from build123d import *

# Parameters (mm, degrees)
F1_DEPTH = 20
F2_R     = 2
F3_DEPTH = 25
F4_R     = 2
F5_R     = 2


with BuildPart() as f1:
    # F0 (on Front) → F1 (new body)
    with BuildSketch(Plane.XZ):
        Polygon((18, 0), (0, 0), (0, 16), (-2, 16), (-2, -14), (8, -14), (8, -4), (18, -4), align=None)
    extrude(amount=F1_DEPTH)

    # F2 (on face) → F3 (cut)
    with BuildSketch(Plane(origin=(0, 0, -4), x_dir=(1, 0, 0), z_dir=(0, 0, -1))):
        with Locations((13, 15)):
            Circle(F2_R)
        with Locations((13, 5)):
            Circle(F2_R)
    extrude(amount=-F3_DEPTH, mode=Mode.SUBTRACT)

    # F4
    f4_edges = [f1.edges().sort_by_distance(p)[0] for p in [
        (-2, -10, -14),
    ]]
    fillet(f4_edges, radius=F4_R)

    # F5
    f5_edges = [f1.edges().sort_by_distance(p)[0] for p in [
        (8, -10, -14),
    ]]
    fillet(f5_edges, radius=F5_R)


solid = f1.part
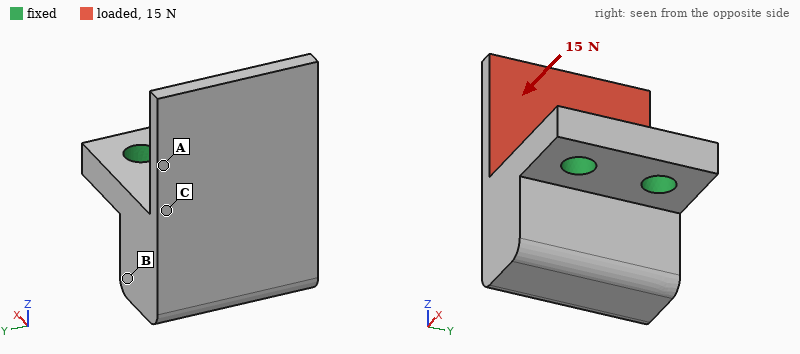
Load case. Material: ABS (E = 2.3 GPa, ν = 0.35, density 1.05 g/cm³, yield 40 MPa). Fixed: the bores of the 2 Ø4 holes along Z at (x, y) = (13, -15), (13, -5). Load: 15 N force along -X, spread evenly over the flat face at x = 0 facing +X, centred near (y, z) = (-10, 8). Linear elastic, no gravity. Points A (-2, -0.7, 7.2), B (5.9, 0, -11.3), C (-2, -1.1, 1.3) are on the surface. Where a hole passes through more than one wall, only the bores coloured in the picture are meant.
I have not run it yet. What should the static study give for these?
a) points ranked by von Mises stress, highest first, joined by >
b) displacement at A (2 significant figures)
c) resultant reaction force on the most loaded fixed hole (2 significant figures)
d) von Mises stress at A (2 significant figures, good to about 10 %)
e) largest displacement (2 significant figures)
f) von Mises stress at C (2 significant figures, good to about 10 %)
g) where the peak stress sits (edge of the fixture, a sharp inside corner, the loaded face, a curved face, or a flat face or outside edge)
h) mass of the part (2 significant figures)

C > A > B
0.15 mm
7.7 N
2.8 MPa
0.38 mm
6.8 MPa
a flat face or outside edge
4.3 g
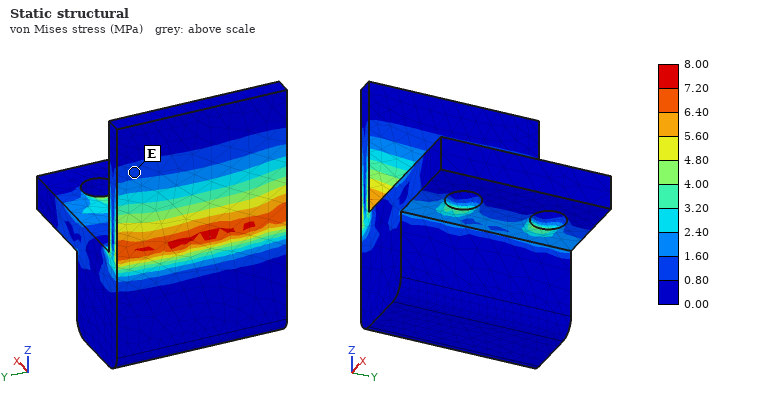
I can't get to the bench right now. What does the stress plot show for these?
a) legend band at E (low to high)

0.80 to 1.60 MPa
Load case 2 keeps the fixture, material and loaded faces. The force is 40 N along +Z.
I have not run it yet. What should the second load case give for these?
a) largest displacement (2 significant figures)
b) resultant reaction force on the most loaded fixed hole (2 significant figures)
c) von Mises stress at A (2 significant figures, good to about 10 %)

0.14 mm
20 N
1.2 MPa
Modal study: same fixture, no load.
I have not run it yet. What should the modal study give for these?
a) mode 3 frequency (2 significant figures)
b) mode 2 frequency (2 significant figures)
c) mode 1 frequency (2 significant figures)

3400 Hz
2200 Hz
1400 Hz
